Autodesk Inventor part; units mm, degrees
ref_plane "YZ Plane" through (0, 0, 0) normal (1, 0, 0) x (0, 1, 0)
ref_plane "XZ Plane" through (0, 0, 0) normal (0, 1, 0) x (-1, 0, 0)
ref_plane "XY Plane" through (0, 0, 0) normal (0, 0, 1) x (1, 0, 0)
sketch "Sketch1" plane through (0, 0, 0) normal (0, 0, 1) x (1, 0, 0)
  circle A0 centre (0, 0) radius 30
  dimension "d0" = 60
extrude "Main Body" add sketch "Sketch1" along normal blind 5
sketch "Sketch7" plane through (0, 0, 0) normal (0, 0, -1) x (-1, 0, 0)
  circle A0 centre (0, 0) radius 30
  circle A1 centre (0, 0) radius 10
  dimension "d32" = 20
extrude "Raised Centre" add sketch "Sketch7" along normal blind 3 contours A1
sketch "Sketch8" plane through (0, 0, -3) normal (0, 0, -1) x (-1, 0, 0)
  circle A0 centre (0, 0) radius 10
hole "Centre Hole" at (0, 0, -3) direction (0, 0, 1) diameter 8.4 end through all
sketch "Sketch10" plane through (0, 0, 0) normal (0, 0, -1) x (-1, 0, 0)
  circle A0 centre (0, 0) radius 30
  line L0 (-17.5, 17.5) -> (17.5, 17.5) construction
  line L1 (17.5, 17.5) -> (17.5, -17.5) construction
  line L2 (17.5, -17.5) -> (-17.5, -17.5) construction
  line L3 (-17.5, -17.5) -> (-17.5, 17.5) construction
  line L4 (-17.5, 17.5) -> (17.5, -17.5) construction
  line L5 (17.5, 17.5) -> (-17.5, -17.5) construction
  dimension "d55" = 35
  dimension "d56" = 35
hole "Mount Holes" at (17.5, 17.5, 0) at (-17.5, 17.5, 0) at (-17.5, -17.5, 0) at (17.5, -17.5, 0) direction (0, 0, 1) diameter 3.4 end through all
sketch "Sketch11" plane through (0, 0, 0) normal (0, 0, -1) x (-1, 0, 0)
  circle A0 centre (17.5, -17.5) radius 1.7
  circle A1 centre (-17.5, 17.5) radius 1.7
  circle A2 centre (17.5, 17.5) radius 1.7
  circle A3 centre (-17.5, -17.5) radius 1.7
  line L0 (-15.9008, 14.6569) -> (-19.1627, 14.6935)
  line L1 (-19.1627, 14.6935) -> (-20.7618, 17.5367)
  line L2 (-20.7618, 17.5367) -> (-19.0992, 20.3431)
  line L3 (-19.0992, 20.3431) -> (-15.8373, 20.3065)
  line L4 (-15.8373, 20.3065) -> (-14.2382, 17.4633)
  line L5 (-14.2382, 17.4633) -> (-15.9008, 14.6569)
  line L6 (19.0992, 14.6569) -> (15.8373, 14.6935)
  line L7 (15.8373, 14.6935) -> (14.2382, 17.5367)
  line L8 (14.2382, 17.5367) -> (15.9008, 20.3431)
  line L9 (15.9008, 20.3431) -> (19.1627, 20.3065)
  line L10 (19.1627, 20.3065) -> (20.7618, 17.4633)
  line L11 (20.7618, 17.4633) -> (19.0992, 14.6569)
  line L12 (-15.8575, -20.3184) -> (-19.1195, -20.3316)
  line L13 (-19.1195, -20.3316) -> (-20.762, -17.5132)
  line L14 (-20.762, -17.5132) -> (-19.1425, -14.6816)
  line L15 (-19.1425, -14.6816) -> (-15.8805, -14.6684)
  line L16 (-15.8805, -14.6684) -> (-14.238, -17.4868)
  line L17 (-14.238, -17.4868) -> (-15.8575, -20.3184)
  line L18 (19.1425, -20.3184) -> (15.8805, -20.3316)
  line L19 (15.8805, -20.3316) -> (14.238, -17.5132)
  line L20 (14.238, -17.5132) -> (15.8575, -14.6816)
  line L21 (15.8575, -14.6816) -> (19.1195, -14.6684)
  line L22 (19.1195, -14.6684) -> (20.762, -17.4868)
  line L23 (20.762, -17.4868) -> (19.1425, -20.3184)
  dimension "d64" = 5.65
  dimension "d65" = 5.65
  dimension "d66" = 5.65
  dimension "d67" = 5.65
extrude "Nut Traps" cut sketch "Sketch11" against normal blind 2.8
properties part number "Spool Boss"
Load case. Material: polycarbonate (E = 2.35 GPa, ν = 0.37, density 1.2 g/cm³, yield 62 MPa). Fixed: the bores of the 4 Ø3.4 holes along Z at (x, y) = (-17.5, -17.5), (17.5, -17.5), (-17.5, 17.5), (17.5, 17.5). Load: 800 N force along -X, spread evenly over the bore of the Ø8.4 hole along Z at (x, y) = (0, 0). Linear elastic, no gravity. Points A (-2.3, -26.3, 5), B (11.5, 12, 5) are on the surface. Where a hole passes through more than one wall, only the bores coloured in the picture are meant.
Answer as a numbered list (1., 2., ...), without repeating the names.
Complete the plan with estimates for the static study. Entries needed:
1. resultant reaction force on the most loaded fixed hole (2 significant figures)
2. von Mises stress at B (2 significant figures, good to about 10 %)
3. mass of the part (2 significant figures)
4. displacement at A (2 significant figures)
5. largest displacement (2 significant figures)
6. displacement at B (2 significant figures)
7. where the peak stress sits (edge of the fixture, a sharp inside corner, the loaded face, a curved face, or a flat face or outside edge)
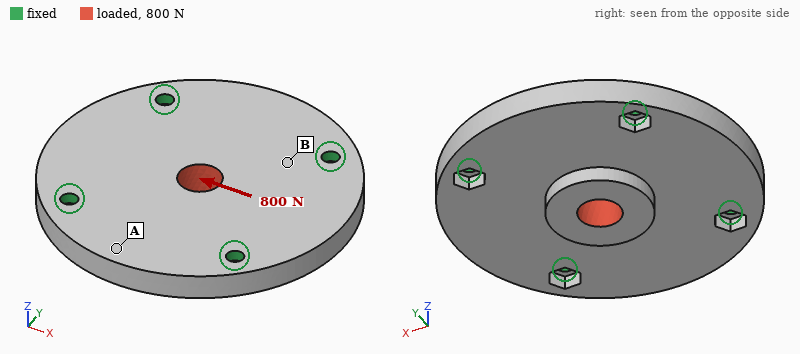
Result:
1. 210 N
2. 4.0 MPa
3. 17 g
4. 13 µm
5. 61 µm
6. 23 µm
7. edge of the fixture
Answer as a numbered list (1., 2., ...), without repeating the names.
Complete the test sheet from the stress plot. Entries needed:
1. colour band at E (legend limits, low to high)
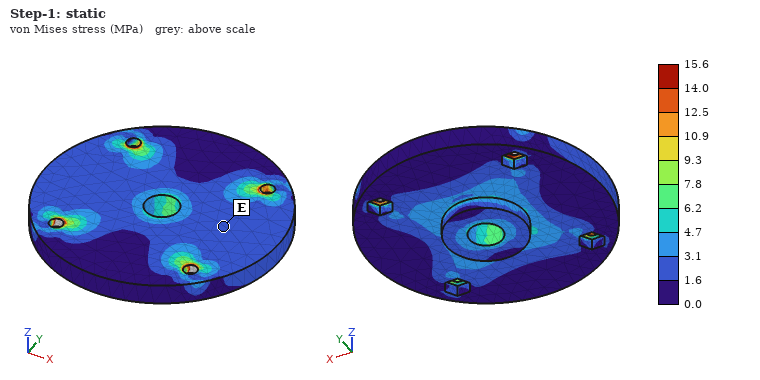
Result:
1. 1.6 to 3.1 MPa
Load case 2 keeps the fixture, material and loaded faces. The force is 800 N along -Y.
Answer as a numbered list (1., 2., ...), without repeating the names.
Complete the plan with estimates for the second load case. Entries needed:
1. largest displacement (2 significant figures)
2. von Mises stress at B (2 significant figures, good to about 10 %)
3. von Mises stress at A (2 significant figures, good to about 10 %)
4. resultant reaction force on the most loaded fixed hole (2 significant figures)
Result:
1. 62 µm
2. 3.9 MPa
3. 2.1 MPa
4. 210 N
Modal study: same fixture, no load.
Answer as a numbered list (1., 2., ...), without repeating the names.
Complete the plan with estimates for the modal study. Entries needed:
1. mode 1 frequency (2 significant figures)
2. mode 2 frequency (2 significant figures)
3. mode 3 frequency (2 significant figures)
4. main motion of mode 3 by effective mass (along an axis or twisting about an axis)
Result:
1. 3100 Hz
2. 3200 Hz
3. 3400 Hz
4. twisting about Y
